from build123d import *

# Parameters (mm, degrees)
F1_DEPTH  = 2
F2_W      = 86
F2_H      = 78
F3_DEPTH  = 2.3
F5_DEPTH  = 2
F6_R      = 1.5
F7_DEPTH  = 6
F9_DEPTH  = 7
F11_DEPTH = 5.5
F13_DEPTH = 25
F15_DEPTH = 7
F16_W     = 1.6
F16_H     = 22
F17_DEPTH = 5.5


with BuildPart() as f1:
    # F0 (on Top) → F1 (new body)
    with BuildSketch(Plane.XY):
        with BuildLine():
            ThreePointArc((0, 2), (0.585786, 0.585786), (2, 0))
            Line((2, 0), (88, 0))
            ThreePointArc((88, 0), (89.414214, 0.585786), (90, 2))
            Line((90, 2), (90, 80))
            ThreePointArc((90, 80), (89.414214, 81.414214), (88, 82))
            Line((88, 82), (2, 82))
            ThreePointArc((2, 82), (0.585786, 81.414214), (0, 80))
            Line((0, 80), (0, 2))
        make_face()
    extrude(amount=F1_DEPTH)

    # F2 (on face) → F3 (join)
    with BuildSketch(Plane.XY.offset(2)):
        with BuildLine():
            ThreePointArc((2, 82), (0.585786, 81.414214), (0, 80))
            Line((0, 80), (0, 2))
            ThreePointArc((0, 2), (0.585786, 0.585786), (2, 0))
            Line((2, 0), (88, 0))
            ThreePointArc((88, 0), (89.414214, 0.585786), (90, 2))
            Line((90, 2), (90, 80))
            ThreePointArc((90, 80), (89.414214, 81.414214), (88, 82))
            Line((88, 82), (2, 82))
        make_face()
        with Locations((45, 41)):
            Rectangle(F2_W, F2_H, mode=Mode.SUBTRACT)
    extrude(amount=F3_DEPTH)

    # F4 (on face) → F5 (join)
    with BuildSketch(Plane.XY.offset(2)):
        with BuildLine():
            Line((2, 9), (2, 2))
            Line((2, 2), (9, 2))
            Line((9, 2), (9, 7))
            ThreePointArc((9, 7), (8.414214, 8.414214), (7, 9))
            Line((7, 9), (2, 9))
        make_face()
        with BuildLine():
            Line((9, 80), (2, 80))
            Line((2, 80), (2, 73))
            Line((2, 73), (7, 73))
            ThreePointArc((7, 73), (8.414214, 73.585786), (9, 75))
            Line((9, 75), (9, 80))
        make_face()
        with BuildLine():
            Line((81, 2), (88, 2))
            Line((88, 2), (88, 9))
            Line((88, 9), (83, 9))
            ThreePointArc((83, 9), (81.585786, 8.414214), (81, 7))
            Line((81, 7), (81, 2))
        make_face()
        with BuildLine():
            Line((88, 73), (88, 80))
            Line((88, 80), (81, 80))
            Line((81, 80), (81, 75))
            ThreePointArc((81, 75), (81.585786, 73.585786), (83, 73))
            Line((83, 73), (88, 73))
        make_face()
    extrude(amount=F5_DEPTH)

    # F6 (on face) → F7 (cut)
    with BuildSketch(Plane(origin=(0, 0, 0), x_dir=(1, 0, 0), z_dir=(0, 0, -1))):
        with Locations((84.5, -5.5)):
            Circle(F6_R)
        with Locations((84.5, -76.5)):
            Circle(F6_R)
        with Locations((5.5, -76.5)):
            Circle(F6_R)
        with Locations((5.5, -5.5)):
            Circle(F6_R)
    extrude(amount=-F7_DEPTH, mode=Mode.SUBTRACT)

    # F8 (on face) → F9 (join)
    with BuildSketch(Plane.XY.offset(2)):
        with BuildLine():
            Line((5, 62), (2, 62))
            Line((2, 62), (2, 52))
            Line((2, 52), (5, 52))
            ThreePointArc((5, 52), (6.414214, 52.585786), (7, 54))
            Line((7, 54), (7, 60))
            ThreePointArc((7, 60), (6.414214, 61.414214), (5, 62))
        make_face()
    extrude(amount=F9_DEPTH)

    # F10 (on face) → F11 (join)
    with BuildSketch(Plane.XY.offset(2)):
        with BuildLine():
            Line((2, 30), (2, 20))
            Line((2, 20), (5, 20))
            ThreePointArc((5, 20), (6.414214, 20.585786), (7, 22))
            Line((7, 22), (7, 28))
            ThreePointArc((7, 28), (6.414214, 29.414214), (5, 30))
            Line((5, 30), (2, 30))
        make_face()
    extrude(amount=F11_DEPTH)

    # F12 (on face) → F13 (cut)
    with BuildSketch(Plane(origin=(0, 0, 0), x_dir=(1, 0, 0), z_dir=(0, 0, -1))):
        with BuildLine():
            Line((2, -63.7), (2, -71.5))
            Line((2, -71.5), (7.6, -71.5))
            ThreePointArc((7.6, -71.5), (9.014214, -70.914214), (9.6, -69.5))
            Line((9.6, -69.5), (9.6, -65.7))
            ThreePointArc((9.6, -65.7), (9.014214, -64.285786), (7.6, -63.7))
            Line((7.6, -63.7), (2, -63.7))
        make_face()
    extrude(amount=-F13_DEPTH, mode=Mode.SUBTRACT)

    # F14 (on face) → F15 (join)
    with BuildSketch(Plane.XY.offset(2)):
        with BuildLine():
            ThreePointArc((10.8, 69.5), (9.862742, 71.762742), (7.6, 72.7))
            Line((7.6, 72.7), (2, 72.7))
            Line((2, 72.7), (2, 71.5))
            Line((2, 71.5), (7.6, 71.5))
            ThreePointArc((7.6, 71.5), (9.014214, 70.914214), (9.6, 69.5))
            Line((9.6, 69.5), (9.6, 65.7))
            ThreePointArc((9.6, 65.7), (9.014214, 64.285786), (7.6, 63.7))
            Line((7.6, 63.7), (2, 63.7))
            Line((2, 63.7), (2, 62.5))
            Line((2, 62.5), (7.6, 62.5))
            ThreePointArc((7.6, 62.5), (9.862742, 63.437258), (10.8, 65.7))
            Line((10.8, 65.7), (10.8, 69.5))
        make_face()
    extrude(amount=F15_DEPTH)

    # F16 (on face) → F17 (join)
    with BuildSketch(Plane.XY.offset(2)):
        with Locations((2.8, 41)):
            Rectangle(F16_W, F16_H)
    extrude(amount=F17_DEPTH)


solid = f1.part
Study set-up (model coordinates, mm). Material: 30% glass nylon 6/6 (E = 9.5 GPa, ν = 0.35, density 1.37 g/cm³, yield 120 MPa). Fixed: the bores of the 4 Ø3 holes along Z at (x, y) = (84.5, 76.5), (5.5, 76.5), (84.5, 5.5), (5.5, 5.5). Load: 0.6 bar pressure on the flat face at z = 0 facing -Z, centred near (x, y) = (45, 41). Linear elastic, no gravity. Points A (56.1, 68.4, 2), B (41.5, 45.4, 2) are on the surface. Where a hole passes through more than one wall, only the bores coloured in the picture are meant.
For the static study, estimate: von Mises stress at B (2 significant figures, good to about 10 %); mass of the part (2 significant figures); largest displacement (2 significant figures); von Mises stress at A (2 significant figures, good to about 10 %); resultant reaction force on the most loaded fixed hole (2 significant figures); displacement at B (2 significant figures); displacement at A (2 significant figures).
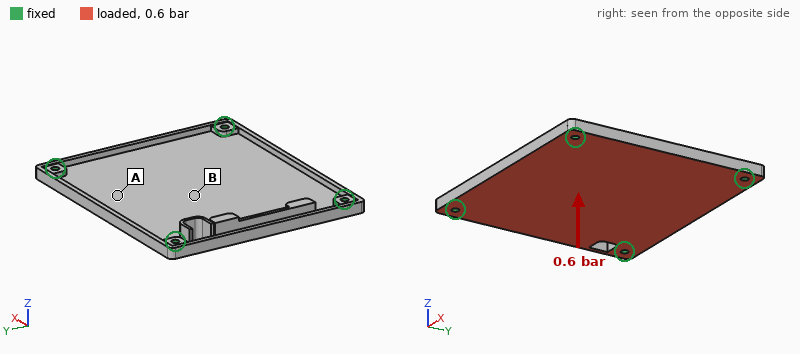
23 MPa
24 g
1.4 mm
13 MPa
140 N
1.3 mm
0.78 mm
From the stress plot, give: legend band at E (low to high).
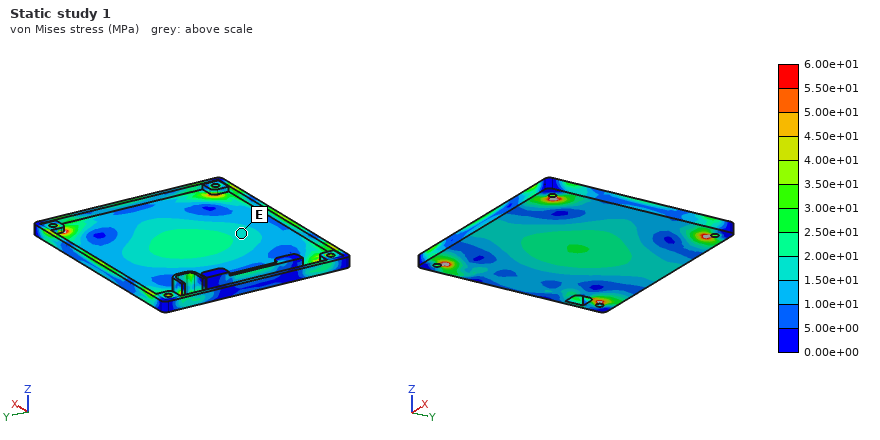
1.50e+01 to 2.00e+01 MPa
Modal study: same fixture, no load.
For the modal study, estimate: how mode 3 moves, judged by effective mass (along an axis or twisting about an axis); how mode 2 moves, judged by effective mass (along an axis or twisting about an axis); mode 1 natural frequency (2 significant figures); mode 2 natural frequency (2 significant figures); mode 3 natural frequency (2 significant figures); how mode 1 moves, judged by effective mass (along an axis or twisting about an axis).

twisting about Y
twisting about X
790 Hz
1400 Hz
1600 Hz
along Z
